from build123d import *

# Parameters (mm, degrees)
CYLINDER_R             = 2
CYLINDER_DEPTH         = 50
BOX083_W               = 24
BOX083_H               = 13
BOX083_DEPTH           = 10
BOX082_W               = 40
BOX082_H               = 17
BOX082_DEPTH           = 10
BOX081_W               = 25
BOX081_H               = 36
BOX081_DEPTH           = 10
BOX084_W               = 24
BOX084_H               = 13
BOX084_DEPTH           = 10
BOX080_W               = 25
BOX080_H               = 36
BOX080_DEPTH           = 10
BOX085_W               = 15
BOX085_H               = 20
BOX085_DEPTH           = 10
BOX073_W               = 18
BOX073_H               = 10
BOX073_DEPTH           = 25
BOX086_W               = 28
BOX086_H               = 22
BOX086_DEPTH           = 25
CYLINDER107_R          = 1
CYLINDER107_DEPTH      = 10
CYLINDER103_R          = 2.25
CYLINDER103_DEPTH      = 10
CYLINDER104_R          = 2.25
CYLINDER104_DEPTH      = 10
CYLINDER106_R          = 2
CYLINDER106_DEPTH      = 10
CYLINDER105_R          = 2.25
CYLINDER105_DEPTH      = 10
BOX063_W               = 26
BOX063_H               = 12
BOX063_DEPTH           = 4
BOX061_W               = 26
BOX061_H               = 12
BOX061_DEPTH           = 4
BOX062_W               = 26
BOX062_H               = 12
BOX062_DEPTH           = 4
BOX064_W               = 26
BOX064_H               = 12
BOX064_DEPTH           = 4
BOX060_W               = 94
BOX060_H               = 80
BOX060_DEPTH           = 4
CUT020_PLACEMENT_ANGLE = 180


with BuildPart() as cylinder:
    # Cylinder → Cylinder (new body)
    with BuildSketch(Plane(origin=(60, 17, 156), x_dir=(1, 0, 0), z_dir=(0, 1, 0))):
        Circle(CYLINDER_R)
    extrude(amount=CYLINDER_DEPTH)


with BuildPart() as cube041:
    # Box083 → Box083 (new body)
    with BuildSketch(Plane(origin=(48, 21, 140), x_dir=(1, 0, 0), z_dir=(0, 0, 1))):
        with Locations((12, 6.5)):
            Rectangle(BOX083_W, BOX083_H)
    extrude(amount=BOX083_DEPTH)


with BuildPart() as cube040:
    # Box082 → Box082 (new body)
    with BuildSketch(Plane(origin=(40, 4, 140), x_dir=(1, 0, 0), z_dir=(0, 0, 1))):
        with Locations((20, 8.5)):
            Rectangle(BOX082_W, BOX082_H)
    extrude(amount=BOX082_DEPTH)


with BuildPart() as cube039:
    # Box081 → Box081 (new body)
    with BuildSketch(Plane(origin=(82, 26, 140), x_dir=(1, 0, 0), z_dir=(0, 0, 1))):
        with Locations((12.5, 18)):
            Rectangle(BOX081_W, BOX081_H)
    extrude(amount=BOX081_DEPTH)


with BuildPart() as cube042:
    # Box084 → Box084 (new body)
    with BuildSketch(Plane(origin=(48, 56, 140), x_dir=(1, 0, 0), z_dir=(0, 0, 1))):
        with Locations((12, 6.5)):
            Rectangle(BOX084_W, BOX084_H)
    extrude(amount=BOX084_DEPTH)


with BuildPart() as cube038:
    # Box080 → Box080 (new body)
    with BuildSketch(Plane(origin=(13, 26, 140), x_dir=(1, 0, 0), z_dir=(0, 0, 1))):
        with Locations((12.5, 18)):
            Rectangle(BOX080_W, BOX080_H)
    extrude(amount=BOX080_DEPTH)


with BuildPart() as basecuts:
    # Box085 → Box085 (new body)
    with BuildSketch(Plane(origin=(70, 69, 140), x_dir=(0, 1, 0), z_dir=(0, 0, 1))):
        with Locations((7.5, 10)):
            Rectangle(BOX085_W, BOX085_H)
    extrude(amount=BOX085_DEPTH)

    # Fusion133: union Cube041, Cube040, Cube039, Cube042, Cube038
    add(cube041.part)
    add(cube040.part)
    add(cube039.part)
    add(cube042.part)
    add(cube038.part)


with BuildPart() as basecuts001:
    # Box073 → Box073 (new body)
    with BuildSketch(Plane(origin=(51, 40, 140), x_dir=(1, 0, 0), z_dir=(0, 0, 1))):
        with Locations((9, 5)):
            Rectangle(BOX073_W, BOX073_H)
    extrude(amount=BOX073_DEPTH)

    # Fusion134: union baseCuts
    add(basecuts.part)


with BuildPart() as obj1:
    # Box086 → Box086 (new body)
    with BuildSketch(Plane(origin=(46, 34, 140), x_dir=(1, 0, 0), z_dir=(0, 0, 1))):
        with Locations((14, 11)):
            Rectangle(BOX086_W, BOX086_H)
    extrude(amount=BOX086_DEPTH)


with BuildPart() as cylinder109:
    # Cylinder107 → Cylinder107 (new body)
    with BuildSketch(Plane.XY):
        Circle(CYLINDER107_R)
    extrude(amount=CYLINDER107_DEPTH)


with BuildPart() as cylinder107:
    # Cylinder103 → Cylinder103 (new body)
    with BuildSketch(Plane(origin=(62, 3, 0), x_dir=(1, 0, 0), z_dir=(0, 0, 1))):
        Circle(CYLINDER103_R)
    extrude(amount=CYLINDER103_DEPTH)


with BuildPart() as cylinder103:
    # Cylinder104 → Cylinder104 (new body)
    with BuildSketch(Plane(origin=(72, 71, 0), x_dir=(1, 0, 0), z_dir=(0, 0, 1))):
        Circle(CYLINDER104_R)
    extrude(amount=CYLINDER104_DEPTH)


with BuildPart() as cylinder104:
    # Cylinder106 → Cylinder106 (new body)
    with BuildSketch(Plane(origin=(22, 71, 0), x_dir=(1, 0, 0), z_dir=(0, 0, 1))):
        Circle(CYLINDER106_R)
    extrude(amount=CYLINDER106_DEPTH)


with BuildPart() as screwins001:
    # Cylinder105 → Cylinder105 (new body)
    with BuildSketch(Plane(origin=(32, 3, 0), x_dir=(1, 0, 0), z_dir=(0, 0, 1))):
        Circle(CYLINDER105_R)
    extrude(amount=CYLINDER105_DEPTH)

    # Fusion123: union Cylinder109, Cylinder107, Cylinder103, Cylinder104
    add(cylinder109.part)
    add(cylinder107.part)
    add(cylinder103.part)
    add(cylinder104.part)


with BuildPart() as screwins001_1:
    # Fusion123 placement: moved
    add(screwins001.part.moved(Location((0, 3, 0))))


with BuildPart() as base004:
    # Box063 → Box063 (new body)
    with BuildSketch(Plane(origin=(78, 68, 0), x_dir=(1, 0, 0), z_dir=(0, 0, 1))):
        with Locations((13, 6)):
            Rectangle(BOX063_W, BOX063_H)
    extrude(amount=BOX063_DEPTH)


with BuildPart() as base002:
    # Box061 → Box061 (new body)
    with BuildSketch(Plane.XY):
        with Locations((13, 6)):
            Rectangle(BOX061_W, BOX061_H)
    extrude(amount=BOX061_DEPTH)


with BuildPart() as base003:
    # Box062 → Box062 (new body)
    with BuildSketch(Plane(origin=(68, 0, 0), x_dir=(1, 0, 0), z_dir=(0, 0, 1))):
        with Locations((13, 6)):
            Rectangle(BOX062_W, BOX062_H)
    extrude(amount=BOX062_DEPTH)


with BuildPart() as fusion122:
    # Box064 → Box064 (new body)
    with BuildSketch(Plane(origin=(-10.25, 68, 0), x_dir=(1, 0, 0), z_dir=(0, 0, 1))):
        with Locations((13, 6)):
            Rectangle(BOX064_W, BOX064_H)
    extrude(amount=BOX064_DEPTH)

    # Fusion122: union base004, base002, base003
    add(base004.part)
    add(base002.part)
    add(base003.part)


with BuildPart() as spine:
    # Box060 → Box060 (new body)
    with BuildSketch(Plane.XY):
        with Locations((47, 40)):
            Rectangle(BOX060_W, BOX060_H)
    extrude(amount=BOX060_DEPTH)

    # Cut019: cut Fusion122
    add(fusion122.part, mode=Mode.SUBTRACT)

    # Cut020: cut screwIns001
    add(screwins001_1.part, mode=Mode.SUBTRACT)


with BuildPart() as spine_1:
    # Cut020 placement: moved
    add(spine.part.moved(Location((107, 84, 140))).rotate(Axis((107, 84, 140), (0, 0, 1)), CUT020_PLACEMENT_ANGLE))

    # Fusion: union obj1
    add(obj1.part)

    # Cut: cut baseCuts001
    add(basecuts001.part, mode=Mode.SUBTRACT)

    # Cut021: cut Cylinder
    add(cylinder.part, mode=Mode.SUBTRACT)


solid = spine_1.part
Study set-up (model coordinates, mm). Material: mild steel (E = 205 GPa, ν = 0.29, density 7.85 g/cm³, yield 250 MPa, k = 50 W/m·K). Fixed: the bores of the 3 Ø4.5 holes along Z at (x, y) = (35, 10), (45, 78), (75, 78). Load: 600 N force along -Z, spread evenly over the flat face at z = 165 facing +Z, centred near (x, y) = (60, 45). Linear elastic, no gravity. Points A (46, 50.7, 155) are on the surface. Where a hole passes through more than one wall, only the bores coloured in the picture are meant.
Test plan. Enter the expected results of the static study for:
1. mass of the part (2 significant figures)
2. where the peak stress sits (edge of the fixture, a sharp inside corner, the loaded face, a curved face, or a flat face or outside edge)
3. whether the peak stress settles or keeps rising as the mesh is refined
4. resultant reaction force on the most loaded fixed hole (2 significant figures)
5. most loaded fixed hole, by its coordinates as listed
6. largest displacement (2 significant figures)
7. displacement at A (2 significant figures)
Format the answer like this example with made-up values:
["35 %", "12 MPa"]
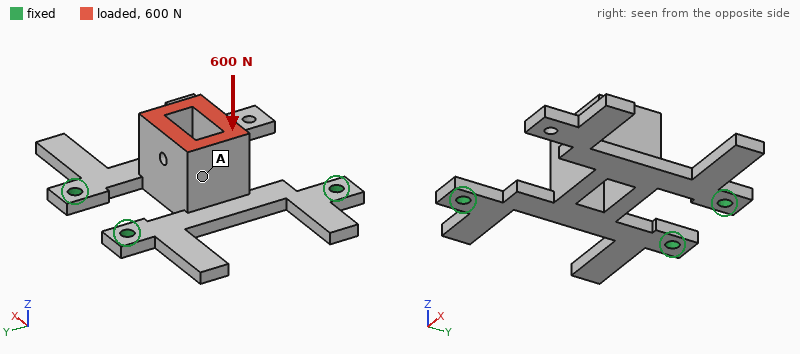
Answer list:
["160 g", "edge of the fixture", "keeps rising", "310 N", "(75, 78)", "0.13 mm", "0.031 mm"]
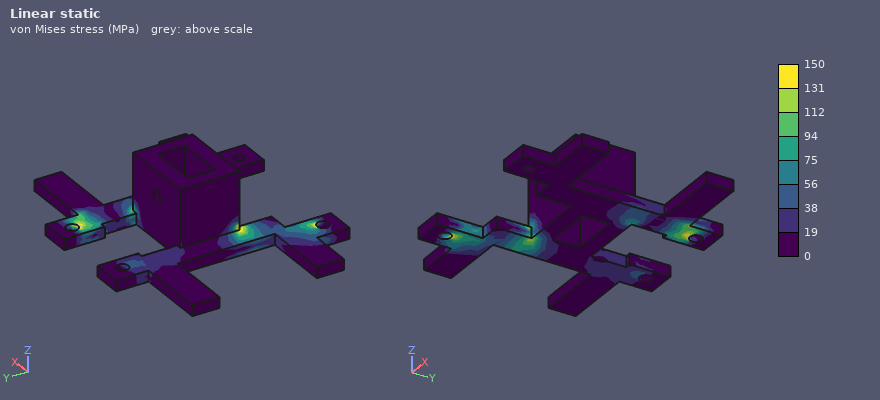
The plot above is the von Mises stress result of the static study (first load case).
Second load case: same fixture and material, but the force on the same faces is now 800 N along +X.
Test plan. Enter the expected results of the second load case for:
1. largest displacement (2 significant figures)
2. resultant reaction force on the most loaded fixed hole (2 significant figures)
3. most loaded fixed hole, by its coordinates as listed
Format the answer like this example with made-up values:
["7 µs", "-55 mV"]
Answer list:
["0.22 mm", "630 N", "(45, 78)"]
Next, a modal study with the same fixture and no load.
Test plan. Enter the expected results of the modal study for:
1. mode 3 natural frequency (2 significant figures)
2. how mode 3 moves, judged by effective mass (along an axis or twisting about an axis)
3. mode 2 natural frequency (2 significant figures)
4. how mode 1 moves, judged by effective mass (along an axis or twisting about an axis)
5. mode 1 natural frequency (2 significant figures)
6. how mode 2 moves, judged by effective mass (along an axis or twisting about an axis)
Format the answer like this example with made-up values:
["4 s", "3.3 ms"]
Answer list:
["2600 Hz", "along X", "2300 Hz", "along Z", "990 Hz", "along Z"]
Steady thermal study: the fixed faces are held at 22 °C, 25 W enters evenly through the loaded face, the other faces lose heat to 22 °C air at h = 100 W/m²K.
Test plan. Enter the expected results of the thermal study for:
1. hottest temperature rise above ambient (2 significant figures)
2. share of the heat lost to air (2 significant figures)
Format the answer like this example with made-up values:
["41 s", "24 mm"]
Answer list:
["47 K", "83 %"]
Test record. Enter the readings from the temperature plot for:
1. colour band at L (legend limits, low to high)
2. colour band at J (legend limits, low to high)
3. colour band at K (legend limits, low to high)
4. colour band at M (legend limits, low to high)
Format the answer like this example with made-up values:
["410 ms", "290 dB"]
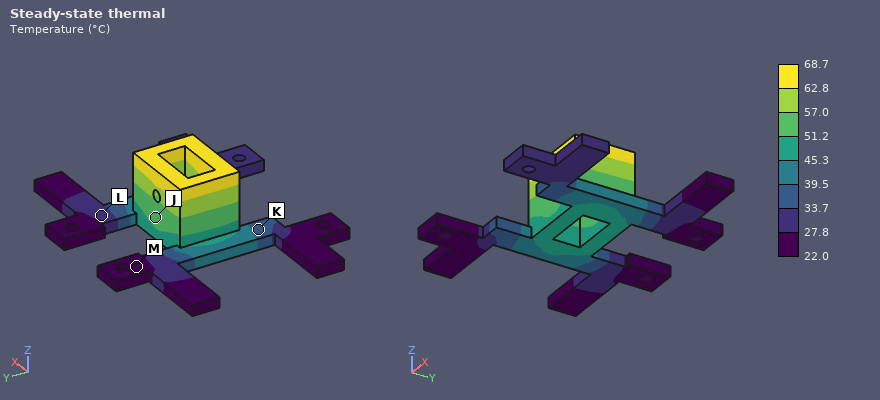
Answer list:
["27.8 to 33.7 °C", "51.2 to 57.0 °C", "33.7 to 39.5 °C", "22.0 to 27.8 °C"]
